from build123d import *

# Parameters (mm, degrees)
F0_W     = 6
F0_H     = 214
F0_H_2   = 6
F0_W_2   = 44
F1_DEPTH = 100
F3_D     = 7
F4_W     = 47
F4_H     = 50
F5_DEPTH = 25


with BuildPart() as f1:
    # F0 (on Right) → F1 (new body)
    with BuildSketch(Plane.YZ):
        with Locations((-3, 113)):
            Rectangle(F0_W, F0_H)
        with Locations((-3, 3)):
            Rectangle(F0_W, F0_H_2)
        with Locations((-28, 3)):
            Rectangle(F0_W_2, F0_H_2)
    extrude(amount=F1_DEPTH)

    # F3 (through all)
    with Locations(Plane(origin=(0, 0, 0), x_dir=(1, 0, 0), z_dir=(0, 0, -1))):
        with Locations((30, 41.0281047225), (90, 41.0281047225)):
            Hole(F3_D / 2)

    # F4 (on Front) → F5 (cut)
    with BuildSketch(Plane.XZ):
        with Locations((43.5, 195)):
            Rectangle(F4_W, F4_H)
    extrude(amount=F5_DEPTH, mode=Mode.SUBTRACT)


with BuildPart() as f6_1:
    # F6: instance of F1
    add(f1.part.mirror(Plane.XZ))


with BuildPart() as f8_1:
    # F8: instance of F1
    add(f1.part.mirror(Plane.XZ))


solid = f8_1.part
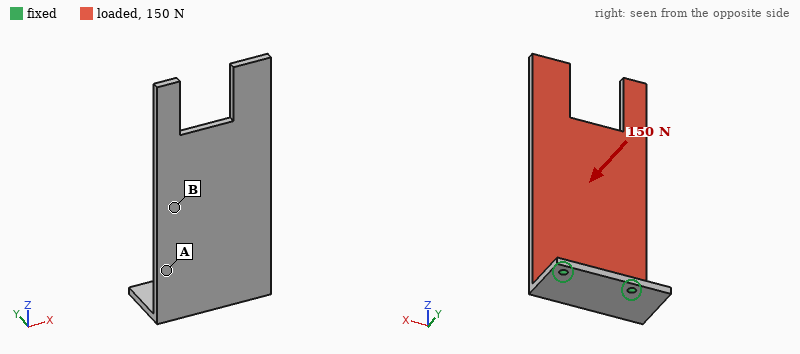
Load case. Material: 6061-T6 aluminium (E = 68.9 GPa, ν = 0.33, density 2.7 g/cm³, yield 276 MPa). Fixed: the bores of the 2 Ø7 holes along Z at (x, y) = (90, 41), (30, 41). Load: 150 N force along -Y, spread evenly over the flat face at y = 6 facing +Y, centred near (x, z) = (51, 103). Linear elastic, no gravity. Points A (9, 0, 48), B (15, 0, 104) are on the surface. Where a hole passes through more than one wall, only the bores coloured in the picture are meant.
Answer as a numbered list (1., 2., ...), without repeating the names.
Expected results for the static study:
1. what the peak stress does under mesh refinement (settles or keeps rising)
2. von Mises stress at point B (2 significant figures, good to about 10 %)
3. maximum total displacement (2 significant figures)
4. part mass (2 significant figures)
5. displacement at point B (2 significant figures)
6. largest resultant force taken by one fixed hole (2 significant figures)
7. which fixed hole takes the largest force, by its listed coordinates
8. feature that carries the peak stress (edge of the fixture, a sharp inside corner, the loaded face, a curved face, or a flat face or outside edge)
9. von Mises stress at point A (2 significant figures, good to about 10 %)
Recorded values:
1. keeps rising
2. 6.0 MPa
3. 2.3 mm
4. 390 g
5. 0.88 mm
6. 110 N
7. (30, 41)
8. edge of the fixture
9. 15 MPa
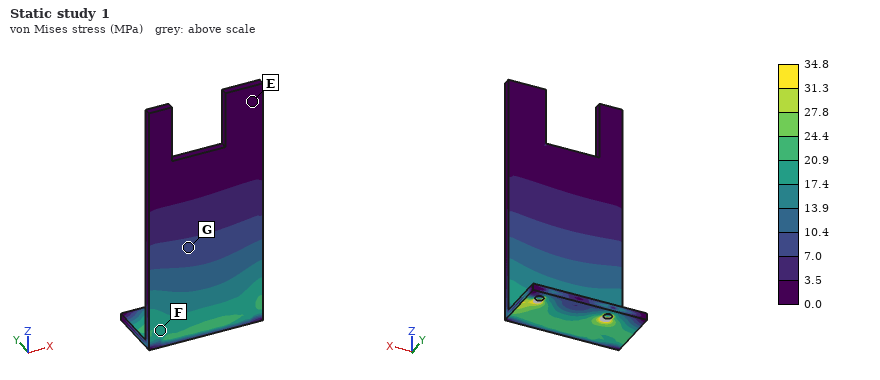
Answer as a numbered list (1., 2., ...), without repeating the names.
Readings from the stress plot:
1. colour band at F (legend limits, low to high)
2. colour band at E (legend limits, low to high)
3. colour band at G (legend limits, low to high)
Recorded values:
1. 17.4 to 20.9 MPa
2. 0.0 to 3.5 MPa
3. 7.0 to 10.4 MPa
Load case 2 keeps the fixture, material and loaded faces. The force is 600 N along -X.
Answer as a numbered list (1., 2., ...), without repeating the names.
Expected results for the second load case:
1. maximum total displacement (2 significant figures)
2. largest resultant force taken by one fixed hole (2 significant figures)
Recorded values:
1. 1.1 mm
2. 1.0 kN
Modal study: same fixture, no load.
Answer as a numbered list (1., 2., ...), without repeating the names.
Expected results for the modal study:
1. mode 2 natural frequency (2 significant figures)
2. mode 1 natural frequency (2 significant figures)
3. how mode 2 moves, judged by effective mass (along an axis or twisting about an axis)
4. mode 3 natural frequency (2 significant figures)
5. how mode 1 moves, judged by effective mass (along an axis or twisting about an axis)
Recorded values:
1. 270 Hz
2. 95 Hz
3. along X
4. 450 Hz
5. along Y
